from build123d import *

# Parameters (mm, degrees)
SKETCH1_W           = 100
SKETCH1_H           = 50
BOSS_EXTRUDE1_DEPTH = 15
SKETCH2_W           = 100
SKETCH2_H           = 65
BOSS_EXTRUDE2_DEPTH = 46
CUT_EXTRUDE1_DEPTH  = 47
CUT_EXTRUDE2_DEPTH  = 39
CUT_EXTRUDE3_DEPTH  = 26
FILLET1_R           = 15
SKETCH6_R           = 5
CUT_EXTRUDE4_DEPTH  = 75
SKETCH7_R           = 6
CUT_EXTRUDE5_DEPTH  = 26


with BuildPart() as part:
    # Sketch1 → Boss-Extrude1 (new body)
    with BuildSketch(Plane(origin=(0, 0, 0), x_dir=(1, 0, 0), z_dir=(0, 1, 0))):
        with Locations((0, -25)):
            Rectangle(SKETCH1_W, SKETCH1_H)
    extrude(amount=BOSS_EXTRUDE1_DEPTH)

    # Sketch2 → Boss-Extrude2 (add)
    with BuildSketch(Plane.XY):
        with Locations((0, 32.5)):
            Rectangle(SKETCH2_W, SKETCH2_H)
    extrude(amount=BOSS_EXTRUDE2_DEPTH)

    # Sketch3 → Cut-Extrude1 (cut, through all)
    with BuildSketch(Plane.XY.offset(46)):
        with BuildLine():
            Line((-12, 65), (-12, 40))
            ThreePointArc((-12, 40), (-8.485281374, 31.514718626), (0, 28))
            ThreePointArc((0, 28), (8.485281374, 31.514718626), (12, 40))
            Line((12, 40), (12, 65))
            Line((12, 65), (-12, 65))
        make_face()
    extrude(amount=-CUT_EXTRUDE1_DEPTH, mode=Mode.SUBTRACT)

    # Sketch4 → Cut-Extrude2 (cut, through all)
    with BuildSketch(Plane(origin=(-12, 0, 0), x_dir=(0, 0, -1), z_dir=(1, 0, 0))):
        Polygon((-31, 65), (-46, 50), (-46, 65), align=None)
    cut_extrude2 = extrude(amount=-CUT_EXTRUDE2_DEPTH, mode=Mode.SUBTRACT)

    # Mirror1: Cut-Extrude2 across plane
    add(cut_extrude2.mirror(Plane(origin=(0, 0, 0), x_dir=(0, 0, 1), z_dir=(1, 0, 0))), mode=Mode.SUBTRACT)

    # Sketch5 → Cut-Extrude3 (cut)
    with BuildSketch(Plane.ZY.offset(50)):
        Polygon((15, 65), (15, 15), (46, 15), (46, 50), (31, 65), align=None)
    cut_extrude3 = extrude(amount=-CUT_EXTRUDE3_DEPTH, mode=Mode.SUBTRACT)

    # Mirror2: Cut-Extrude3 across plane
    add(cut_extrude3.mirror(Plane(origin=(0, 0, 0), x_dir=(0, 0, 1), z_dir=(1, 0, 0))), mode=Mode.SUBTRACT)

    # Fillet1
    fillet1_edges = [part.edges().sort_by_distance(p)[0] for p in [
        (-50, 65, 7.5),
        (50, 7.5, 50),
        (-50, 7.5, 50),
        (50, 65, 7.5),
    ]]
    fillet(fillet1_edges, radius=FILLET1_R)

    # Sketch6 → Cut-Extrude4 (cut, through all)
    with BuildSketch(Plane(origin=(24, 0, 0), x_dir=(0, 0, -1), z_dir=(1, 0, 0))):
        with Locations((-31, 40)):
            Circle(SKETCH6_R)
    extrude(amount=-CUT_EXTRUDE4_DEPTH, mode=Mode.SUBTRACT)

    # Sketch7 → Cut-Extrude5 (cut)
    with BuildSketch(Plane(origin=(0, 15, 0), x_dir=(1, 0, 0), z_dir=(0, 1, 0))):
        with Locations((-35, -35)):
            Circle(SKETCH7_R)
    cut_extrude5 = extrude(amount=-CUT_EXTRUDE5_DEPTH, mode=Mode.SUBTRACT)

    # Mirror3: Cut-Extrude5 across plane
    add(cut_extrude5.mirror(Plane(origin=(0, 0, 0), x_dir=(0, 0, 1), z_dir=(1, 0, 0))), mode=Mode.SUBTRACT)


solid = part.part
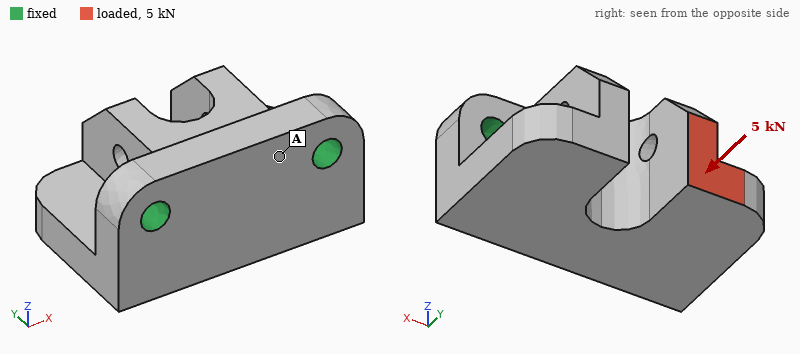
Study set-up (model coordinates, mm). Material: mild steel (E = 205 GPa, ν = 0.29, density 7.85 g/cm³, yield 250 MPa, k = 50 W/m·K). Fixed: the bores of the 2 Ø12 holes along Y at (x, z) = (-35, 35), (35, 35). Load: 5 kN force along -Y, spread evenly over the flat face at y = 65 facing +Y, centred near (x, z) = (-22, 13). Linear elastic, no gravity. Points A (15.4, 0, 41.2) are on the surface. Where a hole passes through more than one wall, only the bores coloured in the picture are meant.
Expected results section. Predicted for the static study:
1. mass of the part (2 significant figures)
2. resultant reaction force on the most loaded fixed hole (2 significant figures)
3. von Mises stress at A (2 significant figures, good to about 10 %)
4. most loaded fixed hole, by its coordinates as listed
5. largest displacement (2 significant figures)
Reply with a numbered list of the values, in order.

1. 1.4 kg
2. 4.2 kN
3. 7.6 MPa
4. (-35, 35)
5. 17 µm
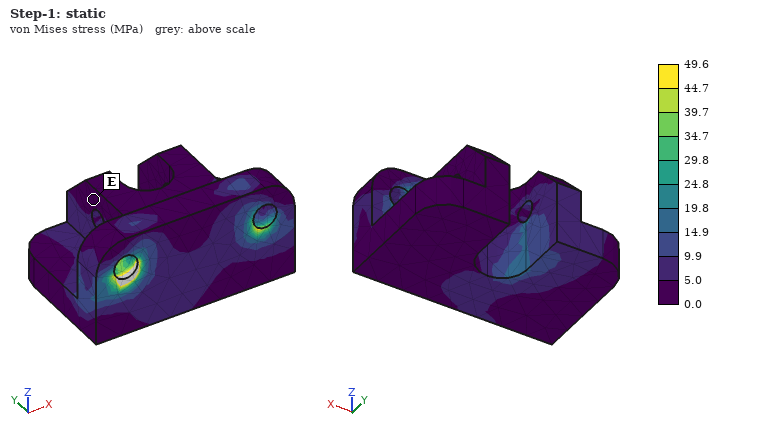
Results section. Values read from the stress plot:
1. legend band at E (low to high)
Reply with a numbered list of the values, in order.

1. 0.0 to 5.0 MPa
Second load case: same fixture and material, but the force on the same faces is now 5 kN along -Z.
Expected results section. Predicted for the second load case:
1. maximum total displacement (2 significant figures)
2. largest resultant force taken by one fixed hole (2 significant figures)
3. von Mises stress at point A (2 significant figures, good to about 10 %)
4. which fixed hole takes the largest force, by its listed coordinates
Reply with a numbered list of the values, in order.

1. 59 µm
2. 4.0 kN
3. 24 MPa
4. (-35, 35)
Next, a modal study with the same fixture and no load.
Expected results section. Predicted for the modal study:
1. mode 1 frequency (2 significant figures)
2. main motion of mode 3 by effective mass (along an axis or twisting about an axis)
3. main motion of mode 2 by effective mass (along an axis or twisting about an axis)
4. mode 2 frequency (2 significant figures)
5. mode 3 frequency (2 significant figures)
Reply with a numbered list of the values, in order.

1. 2900 Hz
2. along X
3. along X
4. 5700 Hz
5. 6800 Hz
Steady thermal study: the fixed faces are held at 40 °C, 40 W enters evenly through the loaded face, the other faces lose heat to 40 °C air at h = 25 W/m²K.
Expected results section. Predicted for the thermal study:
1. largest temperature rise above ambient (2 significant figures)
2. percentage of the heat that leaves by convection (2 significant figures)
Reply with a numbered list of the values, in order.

1. 58 K
2. 21 %
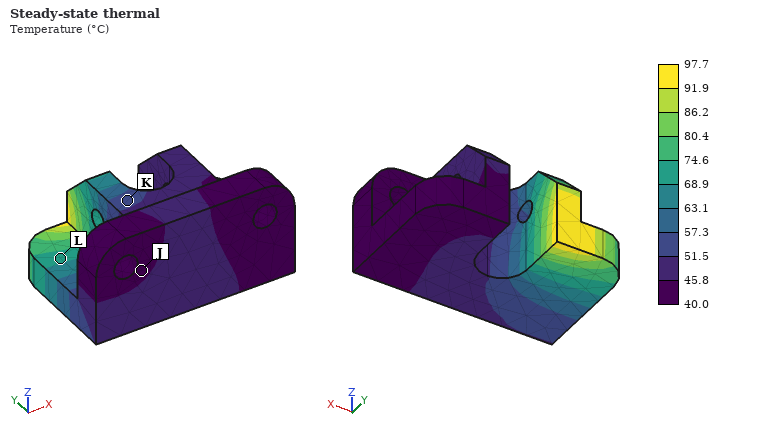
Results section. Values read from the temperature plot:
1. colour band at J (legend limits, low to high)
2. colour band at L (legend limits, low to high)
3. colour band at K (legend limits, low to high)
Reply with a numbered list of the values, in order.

1. 40.0 to 45.8 °C
2. 68.9 to 74.6 °C
3. 51.5 to 57.3 °C
